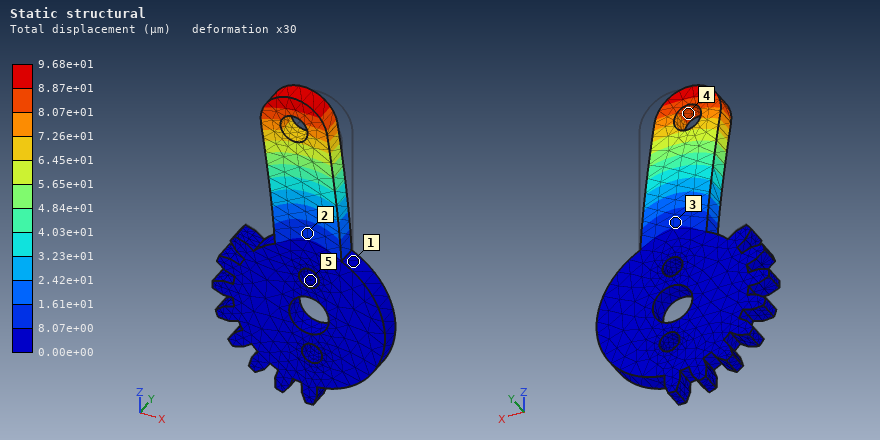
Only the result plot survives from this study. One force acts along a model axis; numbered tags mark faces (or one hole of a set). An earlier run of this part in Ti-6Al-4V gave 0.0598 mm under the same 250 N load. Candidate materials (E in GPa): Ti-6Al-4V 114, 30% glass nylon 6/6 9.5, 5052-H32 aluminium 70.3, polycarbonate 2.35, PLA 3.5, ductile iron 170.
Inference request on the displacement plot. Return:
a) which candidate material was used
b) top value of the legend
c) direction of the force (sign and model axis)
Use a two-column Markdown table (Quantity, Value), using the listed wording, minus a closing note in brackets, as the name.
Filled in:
| Quantity | Value |
|---|---|
| which candidate material was used | 5052-H32 aluminium |
| top value of the legend | 9.68e+01 µm |
| direction of the force | -X |
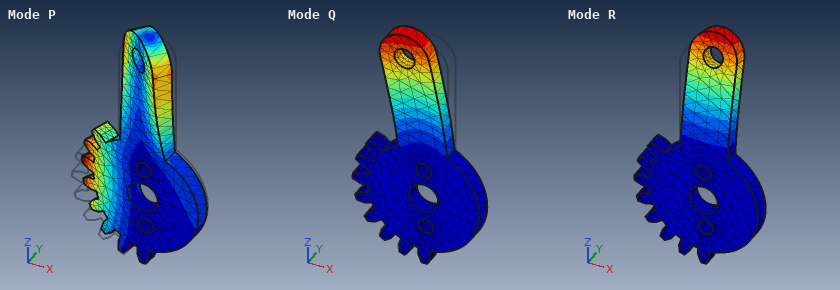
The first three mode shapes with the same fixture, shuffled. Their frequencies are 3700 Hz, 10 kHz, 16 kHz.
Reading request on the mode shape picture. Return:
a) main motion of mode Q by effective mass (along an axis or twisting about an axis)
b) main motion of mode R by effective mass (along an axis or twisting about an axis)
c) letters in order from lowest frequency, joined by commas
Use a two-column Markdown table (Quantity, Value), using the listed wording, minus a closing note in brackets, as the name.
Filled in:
| Quantity | Value |
|---|---|
| main motion of mode Q by effective mass | along X |
| main motion of mode R by effective mass | along Y |
| letters in order from lowest frequency, joined by commas | R, Q, P |
